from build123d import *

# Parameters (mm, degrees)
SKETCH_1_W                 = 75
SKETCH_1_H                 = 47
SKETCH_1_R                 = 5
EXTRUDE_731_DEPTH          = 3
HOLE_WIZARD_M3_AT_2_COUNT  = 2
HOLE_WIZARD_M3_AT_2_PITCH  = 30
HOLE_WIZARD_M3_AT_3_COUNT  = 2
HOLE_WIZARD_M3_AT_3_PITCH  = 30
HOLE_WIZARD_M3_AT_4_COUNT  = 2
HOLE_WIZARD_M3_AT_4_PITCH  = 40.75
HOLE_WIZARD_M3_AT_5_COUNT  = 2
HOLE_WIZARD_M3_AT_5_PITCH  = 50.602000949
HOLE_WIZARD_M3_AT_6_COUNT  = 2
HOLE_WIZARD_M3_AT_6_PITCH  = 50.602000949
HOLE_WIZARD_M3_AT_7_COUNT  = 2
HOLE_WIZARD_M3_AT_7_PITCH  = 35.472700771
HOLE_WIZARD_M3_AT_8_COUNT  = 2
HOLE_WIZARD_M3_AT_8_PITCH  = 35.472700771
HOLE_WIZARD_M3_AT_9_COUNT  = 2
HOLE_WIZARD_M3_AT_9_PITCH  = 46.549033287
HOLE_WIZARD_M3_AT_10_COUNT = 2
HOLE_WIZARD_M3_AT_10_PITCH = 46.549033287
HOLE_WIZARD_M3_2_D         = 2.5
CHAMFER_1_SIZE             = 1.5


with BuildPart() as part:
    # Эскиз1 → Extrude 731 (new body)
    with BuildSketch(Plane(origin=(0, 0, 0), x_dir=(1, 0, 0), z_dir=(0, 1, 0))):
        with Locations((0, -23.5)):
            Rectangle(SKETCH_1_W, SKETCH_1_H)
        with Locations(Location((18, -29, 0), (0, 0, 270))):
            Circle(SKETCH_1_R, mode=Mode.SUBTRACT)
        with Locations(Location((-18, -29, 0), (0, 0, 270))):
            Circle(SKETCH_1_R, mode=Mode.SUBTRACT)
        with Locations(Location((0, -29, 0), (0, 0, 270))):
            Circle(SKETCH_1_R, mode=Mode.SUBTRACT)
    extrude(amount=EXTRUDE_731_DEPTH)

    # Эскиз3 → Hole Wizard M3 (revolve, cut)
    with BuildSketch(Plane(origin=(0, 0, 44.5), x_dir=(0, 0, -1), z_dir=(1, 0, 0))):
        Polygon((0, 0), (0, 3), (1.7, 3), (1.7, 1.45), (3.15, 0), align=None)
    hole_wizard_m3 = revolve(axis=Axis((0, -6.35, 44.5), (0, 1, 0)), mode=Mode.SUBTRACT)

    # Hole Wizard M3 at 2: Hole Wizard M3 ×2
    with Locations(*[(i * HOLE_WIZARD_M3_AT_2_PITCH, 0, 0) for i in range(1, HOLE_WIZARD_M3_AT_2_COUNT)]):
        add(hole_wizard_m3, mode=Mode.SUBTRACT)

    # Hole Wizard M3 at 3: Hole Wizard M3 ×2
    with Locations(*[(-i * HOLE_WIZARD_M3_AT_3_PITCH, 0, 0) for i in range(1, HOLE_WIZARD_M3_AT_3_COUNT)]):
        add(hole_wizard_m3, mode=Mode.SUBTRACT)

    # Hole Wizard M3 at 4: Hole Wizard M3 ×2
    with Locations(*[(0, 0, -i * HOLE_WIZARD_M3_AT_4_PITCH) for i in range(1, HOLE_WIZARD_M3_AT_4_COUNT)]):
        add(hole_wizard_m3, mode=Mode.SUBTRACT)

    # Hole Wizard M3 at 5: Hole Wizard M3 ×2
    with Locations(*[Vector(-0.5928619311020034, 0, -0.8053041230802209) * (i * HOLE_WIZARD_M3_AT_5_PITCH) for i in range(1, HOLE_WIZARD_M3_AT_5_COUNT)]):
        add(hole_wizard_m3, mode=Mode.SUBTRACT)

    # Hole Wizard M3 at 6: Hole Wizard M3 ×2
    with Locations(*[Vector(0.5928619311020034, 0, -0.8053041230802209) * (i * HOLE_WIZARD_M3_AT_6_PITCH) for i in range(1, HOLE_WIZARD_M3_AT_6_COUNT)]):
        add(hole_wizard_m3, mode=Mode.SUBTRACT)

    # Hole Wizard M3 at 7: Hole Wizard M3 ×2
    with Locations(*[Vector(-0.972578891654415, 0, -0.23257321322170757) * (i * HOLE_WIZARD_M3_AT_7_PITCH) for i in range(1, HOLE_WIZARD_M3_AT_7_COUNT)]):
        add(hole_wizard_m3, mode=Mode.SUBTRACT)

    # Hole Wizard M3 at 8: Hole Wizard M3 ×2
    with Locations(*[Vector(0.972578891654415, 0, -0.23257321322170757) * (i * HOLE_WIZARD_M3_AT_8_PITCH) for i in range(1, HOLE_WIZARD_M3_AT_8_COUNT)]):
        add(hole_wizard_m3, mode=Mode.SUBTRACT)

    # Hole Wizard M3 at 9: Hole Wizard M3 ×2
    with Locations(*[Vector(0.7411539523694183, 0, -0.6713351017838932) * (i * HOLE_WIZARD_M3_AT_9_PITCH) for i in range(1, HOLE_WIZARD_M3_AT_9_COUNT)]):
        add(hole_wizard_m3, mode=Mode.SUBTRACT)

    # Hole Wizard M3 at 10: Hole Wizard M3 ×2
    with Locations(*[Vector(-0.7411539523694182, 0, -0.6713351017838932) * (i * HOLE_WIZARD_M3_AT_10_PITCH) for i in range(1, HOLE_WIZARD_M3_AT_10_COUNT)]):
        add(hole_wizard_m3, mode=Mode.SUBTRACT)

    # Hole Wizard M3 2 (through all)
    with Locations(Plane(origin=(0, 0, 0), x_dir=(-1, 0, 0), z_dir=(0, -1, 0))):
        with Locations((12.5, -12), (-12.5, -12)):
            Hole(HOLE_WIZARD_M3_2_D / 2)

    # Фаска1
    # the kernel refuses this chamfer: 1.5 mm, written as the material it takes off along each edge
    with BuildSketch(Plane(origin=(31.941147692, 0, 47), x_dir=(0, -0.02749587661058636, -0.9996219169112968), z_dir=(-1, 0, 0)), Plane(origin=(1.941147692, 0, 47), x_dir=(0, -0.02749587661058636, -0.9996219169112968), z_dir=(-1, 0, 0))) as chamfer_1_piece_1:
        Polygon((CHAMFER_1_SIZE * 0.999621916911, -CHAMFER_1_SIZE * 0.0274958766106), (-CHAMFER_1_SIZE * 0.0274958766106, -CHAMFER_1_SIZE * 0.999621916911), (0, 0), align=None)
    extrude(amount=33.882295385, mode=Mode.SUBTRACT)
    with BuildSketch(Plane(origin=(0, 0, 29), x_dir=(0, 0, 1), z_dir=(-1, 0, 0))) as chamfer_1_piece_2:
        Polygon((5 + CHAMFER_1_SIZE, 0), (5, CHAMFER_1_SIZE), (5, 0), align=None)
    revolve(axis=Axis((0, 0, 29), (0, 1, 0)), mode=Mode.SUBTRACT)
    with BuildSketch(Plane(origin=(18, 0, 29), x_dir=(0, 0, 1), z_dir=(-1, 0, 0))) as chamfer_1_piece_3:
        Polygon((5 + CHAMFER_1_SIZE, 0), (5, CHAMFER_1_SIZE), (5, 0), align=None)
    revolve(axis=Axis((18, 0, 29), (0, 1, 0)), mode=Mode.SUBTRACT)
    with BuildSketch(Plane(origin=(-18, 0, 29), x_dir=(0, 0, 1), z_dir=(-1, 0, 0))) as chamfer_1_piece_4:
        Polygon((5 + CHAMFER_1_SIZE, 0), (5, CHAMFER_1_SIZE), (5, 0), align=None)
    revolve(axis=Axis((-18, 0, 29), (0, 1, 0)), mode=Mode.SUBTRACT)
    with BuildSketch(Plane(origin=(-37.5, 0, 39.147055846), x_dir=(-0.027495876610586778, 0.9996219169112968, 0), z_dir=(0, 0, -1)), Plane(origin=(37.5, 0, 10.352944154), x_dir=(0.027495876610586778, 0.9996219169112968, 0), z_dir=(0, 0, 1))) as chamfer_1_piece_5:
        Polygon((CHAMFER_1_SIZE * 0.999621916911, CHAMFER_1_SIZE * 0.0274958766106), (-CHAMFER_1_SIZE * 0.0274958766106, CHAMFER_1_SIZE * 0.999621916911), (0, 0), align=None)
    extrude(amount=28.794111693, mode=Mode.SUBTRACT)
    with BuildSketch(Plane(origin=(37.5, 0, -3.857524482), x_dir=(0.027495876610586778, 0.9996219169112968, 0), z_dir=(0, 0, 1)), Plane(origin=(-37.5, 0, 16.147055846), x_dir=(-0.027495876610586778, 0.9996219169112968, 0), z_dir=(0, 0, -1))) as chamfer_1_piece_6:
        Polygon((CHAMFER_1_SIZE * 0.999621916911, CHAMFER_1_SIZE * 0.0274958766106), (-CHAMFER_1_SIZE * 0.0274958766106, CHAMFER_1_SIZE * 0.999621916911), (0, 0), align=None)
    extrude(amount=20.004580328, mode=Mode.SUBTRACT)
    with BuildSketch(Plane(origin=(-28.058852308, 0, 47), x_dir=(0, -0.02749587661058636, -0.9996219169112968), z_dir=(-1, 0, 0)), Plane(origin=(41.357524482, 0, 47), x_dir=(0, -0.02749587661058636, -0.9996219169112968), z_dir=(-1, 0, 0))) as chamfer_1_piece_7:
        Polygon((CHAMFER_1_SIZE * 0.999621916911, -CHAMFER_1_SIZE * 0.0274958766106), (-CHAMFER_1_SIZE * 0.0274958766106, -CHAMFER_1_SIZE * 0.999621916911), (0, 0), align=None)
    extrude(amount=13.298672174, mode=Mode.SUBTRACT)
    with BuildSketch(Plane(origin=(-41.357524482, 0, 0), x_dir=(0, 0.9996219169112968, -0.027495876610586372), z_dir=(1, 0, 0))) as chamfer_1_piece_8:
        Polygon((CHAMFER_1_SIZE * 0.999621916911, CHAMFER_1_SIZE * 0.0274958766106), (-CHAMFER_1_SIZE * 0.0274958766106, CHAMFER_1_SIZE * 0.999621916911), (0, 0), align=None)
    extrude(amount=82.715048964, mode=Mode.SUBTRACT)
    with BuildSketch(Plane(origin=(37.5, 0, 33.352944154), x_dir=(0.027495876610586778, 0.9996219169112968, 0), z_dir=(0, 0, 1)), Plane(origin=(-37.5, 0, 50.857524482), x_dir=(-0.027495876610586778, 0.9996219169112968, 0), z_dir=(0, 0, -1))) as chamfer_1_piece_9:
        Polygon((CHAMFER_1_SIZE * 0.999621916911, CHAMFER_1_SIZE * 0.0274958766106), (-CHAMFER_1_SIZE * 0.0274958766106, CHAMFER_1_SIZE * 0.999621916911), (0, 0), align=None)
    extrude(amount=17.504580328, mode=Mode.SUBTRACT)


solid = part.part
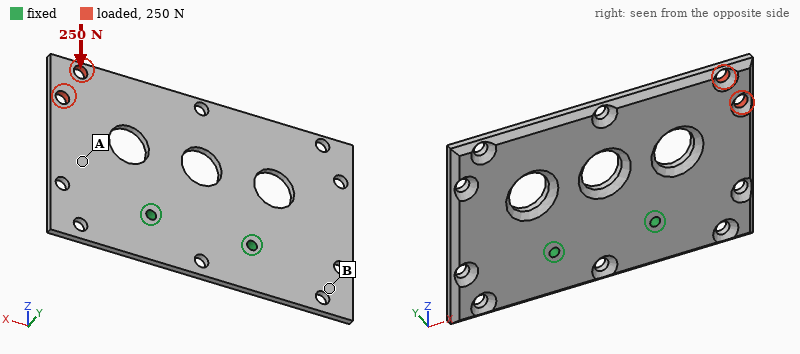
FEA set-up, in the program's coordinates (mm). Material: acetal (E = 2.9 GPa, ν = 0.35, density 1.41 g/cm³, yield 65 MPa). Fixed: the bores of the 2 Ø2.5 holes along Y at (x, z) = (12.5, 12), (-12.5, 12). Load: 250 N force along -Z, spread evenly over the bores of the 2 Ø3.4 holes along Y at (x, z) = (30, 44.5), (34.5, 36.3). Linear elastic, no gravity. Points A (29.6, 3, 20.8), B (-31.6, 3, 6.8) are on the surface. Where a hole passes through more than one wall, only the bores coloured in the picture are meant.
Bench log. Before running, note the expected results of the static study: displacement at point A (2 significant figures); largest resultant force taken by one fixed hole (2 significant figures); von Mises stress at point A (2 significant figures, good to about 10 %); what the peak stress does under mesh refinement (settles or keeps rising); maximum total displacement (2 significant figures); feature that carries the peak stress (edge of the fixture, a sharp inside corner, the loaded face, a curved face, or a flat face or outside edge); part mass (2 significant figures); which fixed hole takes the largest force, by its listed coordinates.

0.18 mm
430 N
7.4 MPa
keeps rising
0.78 mm
edge of the fixture
13 g
(12.5, 12)
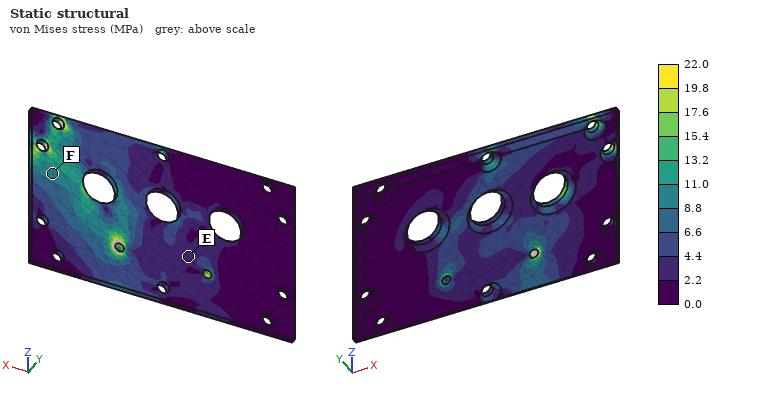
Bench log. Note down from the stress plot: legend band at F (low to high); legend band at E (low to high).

8.8 to 11.0 MPa
2.2 to 4.4 MPa
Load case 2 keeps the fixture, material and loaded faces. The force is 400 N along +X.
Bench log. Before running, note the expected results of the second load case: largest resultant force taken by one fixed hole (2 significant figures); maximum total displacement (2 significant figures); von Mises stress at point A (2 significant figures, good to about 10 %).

470 N
0.99 mm
6.1 MPa
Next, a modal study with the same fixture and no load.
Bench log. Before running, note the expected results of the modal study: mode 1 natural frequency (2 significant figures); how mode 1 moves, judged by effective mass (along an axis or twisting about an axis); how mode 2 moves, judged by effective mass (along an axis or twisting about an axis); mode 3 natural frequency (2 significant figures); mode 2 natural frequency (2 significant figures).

450 Hz
along Y
twisting about Z
910 Hz
570 Hz
